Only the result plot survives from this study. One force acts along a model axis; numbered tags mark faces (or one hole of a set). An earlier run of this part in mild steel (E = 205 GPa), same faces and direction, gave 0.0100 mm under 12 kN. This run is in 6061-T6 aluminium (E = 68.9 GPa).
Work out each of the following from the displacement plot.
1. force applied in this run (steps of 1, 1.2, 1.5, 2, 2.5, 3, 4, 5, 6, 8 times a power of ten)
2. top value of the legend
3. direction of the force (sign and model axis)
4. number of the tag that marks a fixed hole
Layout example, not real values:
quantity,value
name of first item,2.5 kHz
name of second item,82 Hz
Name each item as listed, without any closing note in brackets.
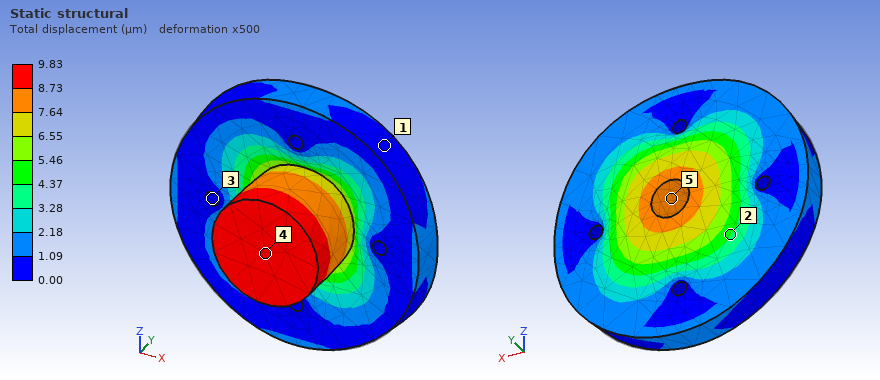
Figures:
quantity,value
force applied in this run,4 kN
top value of the legend,9.83 µm
direction of the force,+Y
number of the tag that marks a fixed hole,3
